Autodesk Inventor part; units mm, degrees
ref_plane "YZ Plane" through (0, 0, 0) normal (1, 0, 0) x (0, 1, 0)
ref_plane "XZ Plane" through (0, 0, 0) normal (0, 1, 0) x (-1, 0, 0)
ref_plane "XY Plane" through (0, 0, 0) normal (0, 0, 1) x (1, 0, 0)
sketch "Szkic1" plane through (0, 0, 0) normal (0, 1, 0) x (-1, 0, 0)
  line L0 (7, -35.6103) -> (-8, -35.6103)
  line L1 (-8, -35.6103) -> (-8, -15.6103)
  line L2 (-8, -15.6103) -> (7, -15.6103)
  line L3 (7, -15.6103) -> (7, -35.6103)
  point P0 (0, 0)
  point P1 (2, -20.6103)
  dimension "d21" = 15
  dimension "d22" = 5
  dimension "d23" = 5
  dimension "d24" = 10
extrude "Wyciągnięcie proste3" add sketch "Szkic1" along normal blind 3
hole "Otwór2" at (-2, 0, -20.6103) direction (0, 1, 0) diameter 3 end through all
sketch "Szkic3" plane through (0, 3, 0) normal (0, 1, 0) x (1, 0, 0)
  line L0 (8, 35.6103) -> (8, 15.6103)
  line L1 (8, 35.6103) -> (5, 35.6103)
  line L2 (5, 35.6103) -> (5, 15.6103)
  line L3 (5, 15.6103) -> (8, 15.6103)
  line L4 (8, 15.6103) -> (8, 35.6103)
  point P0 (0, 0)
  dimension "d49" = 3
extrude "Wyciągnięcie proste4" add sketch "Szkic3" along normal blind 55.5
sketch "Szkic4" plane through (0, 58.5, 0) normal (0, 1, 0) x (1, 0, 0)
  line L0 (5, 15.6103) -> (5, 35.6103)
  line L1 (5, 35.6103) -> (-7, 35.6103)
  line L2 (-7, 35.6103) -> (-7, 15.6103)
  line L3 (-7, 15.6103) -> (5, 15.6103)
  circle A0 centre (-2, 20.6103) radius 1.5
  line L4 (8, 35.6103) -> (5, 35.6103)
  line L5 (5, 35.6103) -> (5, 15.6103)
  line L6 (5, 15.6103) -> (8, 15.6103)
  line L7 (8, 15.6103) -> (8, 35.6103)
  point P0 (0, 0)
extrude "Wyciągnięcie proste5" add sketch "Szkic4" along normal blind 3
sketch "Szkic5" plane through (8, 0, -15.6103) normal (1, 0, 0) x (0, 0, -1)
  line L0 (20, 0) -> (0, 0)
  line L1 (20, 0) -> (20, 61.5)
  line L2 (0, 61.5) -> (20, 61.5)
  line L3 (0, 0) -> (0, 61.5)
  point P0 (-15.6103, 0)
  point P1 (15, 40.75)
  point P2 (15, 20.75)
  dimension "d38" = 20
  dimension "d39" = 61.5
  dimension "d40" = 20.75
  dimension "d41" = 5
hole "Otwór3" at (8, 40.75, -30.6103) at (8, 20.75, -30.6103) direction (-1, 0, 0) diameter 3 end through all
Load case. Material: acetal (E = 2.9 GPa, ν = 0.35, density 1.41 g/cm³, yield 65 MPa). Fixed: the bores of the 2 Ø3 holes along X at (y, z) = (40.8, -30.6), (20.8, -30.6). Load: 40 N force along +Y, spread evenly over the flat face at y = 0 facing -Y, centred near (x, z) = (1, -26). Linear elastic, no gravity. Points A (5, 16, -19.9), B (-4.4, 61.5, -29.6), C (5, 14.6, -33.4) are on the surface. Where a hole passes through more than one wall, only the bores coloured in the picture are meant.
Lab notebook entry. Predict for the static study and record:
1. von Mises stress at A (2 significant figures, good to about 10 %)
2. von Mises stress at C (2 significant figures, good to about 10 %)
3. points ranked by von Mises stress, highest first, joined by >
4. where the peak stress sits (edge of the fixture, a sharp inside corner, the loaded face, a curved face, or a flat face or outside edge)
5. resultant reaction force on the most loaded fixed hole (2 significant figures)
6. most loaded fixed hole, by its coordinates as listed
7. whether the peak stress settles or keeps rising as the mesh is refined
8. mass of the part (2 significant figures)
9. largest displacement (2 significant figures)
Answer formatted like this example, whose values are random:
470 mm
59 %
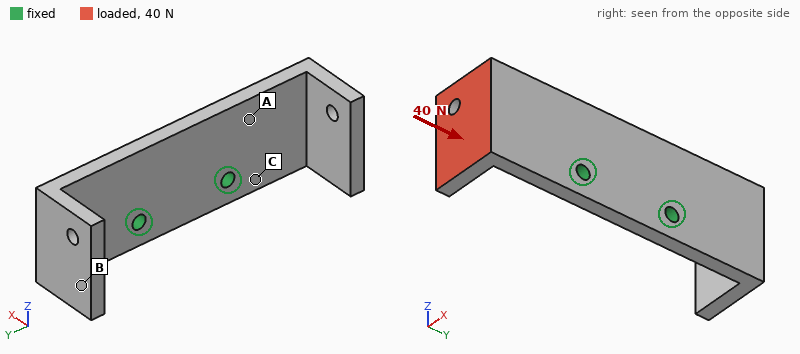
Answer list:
7.0 MPa
9.4 MPa
C > A > B
edge of the fixture
31 N
(20.8, -30.6)
keeps rising
7.1 g
0.69 mm
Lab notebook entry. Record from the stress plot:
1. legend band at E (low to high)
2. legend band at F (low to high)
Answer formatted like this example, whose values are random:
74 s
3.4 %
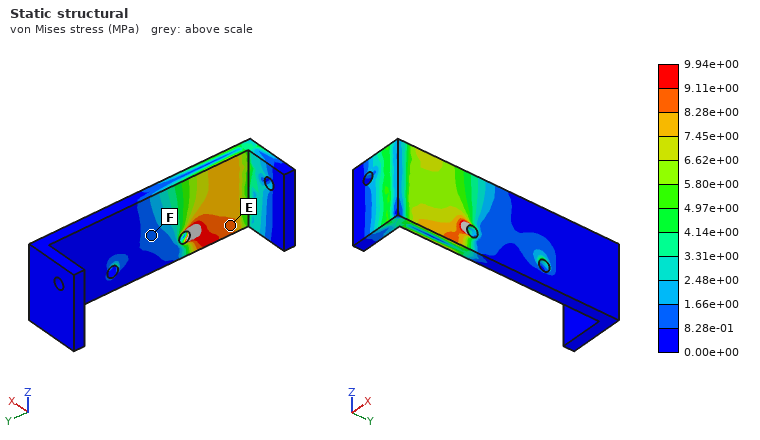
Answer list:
8.28e+00 to 9.11e+00 MPa
8.28e-01 to 1.66e+00 MPa
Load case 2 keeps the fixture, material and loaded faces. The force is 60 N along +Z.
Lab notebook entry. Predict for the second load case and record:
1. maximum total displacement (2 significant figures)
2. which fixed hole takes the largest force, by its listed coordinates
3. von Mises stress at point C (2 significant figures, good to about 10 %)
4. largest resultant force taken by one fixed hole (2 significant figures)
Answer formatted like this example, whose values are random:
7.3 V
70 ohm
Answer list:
0.73 mm
(20.8, -30.6)
12 MPa
120 N
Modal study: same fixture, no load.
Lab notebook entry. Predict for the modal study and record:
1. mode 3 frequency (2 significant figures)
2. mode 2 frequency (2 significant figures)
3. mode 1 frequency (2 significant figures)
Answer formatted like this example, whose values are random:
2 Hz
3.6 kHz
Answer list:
1300 Hz
780 Hz
780 Hz
